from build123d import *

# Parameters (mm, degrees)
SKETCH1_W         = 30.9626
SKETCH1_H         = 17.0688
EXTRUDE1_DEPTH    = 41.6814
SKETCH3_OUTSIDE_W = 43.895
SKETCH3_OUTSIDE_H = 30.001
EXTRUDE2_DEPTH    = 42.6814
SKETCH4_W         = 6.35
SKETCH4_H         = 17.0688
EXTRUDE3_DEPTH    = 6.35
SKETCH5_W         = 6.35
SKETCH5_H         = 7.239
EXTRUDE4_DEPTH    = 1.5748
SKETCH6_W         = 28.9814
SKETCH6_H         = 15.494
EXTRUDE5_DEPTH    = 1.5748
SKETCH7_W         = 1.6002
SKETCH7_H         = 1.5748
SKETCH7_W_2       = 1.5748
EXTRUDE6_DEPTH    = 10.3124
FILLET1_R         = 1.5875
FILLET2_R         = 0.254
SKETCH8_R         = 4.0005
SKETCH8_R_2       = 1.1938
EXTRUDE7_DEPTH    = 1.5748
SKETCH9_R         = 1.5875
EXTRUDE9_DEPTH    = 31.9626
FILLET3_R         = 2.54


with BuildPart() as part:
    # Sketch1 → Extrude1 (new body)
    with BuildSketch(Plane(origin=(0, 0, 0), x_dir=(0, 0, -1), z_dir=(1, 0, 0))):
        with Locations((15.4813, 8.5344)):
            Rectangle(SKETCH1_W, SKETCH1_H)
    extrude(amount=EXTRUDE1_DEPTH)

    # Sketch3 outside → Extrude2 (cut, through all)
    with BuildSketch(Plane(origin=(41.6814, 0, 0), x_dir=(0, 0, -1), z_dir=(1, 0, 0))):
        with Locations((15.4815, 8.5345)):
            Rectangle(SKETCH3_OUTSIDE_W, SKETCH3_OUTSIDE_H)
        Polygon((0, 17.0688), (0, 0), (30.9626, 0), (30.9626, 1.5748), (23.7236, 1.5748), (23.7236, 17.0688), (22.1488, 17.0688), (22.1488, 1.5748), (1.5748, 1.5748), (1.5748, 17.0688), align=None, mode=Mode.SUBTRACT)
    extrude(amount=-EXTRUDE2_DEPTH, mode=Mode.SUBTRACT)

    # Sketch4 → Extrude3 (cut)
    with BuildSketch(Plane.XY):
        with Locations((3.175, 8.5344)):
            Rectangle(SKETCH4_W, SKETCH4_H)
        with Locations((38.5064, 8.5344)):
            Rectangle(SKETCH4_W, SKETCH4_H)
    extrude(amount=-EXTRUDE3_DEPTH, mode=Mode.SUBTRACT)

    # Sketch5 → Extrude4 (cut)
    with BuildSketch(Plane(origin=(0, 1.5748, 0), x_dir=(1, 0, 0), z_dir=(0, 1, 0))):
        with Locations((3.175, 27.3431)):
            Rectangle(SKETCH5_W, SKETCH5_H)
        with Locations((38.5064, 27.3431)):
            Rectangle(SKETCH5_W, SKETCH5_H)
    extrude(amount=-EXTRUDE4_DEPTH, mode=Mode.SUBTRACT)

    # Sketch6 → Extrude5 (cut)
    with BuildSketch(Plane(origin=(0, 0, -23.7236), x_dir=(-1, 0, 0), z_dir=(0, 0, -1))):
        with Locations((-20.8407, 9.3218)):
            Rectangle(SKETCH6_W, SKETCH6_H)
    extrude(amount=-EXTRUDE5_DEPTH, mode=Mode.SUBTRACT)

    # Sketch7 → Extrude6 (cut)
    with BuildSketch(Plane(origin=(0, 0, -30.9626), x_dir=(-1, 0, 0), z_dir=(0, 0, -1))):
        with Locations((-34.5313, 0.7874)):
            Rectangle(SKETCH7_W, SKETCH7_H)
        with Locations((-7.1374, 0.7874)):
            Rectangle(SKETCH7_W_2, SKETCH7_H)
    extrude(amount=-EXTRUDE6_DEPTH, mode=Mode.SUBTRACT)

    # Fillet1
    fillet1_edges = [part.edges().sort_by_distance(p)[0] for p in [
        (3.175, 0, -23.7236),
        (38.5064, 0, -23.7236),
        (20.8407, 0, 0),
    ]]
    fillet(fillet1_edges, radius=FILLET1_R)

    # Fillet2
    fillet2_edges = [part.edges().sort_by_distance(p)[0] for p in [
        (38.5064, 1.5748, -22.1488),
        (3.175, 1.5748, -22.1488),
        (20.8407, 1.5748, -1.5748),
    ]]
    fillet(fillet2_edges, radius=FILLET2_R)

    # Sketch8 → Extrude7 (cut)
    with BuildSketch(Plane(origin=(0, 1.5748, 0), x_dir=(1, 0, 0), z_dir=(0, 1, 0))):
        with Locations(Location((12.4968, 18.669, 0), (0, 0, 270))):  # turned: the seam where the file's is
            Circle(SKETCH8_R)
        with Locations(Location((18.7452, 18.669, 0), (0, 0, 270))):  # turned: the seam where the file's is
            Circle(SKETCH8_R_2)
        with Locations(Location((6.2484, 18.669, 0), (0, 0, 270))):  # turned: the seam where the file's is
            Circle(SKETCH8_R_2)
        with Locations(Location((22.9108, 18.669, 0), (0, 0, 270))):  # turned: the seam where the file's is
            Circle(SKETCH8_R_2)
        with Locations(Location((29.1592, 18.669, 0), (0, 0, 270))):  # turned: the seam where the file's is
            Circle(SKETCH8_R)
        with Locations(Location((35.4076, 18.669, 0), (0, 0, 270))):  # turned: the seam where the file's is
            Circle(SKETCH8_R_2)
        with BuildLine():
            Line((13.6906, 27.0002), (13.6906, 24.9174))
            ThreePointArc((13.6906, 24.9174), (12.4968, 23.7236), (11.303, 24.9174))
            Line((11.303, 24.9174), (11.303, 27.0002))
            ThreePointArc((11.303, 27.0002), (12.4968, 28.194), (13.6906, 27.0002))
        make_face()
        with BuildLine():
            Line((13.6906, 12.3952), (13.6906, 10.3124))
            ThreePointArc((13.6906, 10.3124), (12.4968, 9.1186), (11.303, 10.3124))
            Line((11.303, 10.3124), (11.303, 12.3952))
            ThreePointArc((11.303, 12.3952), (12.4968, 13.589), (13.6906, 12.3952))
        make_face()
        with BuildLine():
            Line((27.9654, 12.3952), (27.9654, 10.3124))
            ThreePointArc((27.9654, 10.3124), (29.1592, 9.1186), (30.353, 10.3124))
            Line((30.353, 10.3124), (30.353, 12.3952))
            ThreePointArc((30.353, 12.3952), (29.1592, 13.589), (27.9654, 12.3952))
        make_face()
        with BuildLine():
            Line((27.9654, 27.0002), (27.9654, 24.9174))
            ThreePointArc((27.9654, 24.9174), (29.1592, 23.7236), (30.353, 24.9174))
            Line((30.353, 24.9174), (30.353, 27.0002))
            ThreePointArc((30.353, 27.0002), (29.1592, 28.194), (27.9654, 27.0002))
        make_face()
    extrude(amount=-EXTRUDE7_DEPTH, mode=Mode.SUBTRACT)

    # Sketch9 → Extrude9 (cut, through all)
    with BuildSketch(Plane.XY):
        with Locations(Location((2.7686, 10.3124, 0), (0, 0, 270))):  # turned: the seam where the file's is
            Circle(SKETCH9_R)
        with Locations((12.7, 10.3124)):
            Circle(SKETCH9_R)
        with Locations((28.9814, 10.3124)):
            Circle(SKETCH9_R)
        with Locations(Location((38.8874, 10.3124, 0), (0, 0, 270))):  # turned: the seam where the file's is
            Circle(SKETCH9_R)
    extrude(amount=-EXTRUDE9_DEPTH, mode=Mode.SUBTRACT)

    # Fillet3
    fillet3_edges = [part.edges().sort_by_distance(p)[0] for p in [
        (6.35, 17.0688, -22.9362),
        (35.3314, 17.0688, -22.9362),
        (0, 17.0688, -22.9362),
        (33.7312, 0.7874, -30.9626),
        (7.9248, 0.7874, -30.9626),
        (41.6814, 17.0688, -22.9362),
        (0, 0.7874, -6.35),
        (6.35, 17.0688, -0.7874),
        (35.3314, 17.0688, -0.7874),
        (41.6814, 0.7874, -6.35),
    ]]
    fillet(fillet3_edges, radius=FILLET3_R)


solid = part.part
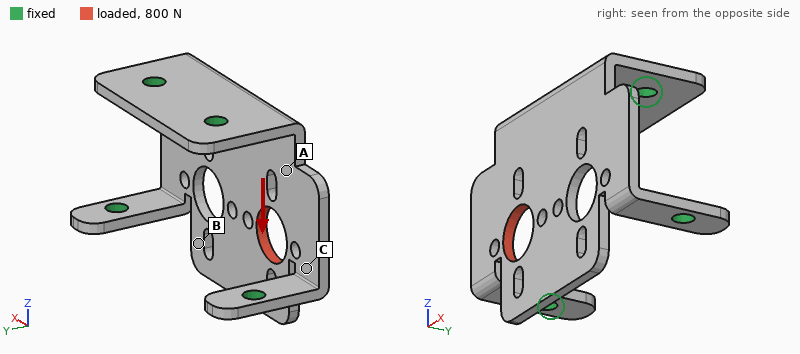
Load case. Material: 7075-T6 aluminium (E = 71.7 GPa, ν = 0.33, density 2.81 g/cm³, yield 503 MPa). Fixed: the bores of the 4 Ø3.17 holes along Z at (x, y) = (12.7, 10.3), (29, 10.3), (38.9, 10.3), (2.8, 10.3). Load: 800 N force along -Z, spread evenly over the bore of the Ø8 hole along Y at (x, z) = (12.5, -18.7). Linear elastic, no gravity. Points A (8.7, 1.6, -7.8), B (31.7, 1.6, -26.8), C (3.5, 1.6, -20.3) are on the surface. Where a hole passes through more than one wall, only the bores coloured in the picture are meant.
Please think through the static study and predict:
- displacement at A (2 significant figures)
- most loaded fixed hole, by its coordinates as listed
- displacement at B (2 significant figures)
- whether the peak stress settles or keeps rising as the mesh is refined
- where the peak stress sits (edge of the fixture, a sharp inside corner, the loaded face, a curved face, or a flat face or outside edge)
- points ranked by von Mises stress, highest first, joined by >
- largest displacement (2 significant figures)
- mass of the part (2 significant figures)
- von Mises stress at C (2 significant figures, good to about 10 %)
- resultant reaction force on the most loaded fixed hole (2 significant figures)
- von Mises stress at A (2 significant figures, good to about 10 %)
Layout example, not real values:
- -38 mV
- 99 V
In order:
- 0.12 mm
- (12.7, 10.3)
- 0.088 mm
- keeps rising
- edge of the fixture
- C > A > B
- 0.14 mm
- 6.7 g
- 180 MPa
- 310 N
- 96 MPa
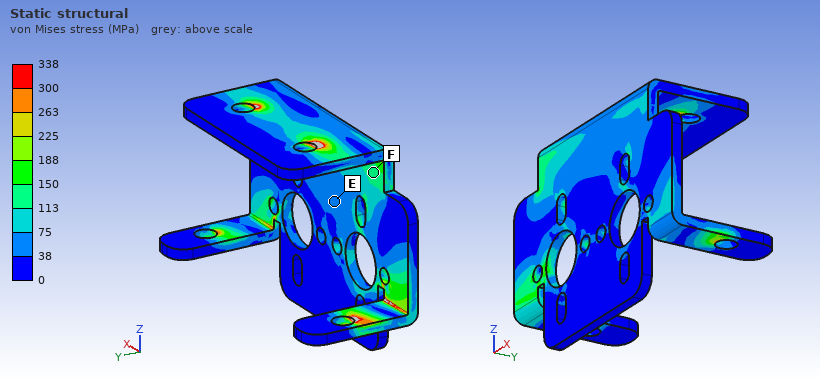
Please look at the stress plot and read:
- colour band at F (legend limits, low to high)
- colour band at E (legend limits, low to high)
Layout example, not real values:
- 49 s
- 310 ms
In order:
- 113 to 150 MPa
- 38 to 75 MPa
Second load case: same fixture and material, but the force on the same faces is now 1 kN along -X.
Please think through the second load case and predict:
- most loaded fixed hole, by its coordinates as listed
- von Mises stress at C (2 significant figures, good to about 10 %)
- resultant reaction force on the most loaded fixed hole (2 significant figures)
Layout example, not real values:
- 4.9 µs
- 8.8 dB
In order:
- (2.8, 10.3)
- 110 MPa
- 350 N
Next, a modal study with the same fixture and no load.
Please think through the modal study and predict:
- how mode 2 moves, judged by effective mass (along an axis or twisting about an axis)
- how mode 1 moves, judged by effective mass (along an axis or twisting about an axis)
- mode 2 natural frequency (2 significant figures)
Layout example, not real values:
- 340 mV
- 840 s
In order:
- along Z
- along Y
- 6600 Hz
